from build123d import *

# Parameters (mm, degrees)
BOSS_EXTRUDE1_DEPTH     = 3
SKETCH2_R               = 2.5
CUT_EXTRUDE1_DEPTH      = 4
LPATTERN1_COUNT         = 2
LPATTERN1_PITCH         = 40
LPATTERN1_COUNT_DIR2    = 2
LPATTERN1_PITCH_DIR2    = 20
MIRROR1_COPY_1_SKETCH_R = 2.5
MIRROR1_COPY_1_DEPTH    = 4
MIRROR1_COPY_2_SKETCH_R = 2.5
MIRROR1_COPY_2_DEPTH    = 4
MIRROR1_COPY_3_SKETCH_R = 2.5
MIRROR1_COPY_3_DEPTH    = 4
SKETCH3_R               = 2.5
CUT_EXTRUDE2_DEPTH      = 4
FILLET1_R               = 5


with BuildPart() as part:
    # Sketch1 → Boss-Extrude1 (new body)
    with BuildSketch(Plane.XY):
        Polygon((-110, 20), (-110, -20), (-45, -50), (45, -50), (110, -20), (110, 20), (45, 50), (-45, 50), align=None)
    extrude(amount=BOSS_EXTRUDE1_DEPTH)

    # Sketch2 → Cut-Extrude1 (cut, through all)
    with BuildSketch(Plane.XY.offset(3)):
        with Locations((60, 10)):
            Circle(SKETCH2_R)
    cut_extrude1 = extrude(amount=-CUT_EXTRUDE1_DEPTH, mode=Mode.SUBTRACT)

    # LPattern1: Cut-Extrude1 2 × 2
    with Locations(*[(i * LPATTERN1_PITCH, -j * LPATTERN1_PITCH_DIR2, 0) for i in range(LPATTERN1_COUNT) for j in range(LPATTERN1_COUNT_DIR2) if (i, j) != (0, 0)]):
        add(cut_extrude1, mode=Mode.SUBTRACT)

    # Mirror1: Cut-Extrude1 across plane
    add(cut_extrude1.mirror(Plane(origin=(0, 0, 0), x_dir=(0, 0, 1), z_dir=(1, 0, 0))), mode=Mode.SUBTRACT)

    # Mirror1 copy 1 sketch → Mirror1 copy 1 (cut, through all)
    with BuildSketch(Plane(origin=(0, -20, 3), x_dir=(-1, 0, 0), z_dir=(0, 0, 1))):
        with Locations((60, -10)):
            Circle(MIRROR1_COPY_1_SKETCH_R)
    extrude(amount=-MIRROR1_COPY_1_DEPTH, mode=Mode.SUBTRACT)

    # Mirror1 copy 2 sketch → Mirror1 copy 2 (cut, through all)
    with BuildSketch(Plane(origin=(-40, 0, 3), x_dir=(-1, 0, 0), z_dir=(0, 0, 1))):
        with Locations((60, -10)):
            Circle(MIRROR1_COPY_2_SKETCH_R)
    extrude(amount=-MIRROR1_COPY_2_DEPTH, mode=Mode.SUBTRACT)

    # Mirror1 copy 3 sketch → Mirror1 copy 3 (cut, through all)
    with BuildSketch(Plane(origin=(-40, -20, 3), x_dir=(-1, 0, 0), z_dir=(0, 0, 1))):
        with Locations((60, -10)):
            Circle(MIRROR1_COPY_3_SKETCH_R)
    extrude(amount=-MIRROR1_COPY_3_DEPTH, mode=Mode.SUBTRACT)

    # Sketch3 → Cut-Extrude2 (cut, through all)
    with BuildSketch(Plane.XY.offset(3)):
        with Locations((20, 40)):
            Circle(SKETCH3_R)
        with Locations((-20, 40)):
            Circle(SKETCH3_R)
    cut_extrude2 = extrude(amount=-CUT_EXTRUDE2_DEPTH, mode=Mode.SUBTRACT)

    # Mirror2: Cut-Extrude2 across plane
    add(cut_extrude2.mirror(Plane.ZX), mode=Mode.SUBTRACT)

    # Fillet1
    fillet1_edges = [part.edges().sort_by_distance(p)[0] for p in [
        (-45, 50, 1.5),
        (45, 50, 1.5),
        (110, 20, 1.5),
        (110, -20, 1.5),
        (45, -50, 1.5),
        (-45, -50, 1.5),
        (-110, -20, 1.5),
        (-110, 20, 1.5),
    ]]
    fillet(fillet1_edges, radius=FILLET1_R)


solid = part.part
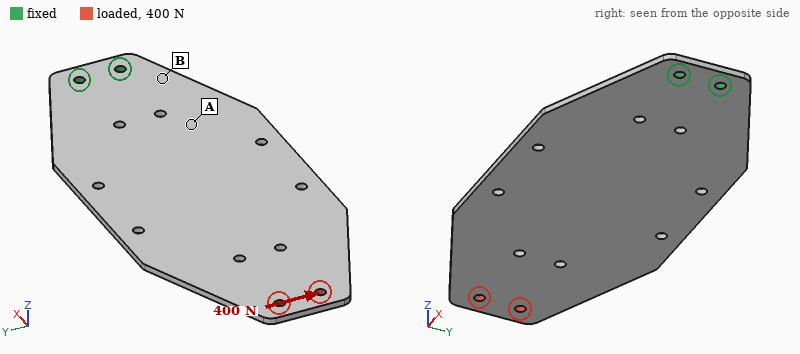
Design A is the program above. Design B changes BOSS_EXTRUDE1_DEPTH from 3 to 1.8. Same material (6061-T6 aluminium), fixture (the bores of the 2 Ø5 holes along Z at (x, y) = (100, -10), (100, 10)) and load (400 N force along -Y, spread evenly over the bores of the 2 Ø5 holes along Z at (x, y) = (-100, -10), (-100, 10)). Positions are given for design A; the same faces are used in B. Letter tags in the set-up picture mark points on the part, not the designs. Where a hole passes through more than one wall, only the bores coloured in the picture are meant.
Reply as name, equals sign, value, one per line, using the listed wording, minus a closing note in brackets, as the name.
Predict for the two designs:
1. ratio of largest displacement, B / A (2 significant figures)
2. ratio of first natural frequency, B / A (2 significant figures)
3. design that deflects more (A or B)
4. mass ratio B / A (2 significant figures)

ratio of largest displacement, B / A = 1.7
ratio of first natural frequency, B / A = 0.60
design that deflects more = B
mass ratio B / A = 0.60
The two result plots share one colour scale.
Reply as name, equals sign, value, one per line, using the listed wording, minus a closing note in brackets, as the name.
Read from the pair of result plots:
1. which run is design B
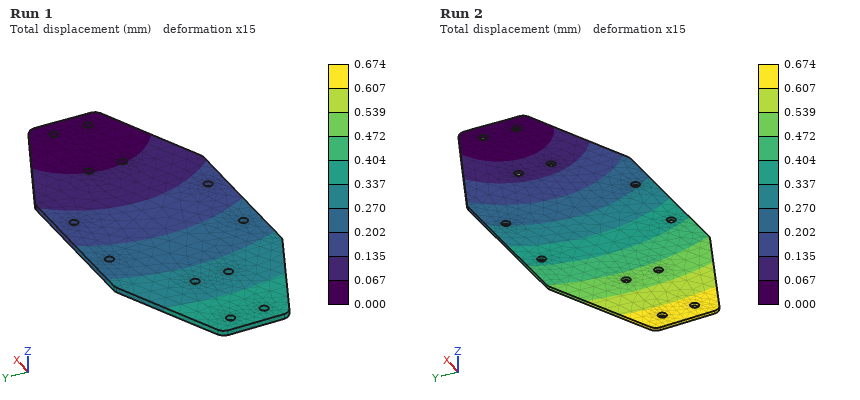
which run is design B = Run 2
